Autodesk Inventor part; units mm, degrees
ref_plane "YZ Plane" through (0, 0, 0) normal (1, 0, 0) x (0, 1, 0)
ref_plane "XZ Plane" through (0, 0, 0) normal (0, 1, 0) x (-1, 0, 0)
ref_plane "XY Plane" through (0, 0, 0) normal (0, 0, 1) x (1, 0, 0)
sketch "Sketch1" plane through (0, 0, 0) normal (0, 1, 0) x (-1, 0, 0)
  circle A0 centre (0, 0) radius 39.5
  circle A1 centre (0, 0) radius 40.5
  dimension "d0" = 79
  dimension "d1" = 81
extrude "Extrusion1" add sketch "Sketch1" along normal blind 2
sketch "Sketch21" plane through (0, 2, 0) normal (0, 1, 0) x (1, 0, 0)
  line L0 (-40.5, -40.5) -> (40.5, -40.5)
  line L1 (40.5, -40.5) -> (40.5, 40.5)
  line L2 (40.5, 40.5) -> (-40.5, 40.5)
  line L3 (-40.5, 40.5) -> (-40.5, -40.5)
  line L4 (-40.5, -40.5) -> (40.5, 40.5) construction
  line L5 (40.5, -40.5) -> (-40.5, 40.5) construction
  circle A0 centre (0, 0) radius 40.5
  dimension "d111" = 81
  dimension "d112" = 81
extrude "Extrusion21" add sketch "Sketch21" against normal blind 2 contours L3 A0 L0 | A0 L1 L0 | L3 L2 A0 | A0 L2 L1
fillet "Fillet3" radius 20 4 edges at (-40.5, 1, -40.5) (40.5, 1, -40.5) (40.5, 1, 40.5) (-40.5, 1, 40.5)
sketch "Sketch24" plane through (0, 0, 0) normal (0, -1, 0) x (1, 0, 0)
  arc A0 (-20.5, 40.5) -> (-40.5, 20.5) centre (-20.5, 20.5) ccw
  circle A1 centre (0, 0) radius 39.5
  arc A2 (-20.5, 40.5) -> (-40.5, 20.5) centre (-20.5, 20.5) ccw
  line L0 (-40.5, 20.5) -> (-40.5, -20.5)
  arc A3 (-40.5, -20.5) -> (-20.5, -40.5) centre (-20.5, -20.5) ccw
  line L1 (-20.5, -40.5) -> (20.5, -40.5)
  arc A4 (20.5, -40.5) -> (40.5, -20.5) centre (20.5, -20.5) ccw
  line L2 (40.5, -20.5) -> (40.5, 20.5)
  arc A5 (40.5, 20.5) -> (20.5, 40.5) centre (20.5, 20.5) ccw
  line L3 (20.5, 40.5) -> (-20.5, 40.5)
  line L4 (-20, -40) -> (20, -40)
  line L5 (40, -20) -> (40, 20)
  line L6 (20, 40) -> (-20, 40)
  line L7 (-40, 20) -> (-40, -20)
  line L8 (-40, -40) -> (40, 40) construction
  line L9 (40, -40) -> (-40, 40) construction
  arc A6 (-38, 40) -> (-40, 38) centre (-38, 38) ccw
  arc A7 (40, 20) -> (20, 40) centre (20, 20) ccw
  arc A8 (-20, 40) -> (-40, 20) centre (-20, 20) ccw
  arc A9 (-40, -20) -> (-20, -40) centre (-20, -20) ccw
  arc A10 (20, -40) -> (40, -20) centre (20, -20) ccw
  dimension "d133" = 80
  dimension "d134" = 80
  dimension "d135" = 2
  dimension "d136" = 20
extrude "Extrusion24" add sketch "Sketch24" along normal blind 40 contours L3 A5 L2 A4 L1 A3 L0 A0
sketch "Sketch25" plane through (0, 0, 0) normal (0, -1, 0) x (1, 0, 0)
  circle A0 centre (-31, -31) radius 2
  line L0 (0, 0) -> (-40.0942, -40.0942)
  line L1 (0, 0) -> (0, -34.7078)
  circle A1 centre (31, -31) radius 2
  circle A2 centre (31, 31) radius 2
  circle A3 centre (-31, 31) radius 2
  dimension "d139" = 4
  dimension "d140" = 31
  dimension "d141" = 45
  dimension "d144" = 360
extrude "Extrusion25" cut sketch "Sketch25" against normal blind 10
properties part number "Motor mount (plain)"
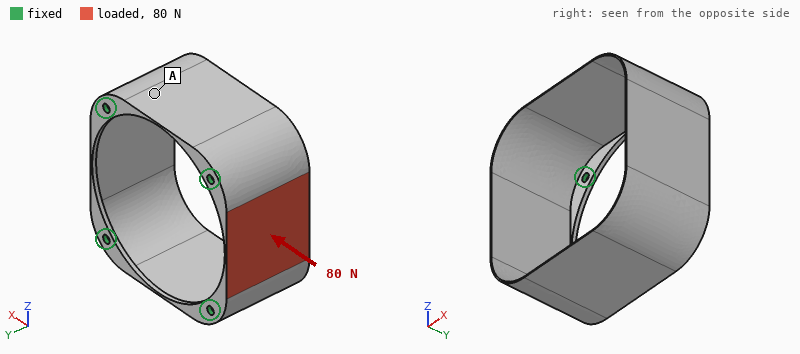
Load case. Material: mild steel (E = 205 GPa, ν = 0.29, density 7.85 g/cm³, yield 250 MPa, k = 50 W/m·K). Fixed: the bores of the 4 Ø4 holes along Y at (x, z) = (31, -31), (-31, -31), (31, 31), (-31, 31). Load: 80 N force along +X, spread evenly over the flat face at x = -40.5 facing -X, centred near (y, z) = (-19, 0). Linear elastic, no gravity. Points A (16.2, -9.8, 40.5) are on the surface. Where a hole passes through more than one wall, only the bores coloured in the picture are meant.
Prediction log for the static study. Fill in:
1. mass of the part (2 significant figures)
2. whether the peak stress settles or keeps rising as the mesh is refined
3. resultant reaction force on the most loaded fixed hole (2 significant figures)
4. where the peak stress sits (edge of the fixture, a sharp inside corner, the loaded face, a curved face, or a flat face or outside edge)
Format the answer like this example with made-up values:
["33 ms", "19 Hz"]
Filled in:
["70 g", "keeps rising", "77 N", "edge of the fixture"]
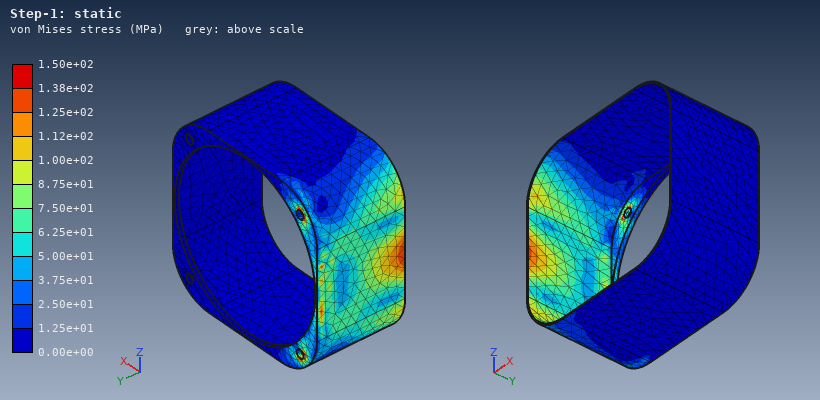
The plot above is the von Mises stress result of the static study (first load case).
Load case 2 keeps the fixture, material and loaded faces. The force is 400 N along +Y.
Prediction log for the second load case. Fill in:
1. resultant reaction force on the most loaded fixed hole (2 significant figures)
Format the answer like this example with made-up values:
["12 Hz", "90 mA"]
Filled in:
["210 N"]
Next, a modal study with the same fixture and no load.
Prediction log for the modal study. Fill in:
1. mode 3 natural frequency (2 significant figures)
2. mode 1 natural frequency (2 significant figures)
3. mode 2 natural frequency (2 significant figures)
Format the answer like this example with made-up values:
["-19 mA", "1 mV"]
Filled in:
["840 Hz", "780 Hz", "840 Hz"]
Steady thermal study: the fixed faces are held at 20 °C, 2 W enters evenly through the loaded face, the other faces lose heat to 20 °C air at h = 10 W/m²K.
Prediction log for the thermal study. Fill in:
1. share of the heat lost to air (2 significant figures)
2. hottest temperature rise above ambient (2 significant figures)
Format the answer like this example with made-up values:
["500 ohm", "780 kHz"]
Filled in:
["36 %", "20 K"]
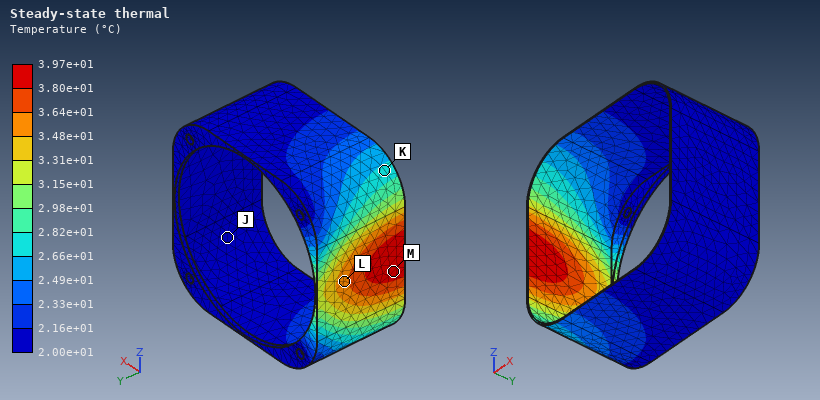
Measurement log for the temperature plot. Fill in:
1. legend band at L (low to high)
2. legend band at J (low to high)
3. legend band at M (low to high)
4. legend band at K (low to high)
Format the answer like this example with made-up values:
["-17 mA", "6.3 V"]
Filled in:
["3.48e+01 to 3.64e+01 °C", "2.00e+01 to 2.16e+01 °C", "3.80e+01 to 3.97e+01 °C", "2.66e+01 to 2.82e+01 °C"]
